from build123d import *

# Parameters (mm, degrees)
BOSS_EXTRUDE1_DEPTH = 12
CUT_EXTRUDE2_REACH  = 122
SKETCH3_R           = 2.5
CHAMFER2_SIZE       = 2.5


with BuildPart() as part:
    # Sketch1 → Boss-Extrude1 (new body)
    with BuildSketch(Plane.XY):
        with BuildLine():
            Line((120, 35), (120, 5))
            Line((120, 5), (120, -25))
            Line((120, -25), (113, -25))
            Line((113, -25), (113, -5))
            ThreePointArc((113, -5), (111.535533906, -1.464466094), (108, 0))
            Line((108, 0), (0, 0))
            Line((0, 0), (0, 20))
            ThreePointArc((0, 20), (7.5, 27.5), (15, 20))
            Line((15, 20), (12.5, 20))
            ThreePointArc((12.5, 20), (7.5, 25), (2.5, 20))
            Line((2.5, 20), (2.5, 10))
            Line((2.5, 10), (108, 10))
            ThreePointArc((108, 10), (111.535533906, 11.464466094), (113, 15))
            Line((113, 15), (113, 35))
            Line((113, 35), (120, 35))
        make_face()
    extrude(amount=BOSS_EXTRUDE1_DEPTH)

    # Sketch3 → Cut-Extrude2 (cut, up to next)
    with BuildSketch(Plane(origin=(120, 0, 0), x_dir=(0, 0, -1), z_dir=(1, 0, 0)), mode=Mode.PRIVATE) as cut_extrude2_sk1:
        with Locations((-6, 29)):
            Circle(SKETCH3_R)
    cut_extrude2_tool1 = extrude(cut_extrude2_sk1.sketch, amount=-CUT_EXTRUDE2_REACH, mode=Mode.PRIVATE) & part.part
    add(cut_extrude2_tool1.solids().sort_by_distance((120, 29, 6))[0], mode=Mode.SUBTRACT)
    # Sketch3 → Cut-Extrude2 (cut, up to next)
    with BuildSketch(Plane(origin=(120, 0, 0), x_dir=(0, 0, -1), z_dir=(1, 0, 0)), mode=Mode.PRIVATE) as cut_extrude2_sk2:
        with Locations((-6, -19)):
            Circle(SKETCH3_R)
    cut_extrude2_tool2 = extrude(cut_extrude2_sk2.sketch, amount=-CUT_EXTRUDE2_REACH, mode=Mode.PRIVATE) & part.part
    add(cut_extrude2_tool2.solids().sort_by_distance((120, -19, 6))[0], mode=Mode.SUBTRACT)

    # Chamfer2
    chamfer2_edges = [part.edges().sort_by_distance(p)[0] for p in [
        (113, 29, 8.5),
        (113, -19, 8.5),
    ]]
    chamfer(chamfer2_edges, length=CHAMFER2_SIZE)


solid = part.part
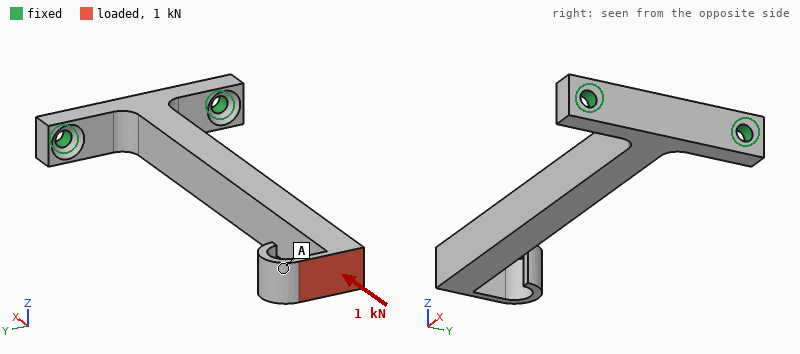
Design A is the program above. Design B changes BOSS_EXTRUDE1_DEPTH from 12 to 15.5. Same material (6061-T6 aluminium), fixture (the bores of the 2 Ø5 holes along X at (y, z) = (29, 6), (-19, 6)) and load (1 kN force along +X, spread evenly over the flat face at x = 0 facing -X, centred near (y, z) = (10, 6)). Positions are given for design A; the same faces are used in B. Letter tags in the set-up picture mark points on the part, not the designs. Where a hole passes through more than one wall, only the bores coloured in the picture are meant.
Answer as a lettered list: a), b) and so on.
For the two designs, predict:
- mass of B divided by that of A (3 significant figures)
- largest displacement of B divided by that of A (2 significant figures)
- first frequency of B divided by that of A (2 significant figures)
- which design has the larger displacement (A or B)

a) 1.30
b) 0.78
c) 1.1
d) A
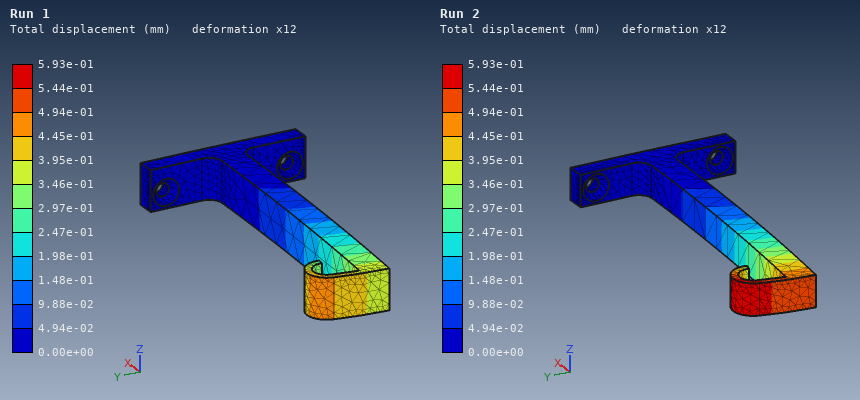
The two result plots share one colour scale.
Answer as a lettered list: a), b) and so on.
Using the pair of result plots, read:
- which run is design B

a) Run 1
